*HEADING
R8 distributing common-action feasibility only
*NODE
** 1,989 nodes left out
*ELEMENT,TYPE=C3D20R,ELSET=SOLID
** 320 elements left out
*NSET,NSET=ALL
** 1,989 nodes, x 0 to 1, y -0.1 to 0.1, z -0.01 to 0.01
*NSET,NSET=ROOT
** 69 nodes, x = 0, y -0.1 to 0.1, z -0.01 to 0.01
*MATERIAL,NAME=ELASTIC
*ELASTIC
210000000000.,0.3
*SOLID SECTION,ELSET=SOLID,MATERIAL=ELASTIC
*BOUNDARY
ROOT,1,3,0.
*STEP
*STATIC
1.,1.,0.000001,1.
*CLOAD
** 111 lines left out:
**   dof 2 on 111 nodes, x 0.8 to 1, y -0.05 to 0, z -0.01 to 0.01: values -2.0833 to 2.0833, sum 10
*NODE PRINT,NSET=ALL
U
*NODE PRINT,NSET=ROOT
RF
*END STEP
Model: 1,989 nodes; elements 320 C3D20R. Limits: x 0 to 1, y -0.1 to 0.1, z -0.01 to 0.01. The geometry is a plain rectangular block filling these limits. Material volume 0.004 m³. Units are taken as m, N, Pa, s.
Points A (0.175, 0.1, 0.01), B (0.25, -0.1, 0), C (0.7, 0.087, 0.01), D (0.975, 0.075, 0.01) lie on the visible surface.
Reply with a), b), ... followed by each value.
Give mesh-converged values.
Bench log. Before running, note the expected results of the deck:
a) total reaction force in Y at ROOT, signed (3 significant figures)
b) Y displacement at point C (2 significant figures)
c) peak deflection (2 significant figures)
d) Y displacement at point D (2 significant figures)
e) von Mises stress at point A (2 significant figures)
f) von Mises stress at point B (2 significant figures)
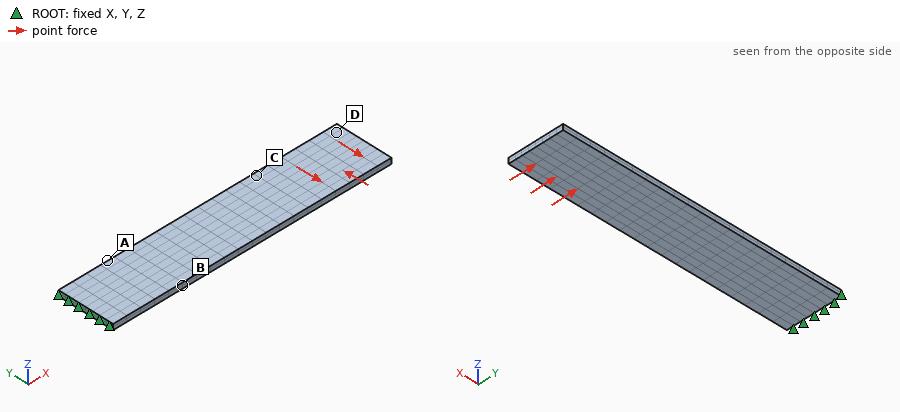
a) -10.0 N
b) 6.9e-07 m
c) 1.6e-06 m
d) 1.1e-06 m
e) 53000 Pa
f) 54000 Pa
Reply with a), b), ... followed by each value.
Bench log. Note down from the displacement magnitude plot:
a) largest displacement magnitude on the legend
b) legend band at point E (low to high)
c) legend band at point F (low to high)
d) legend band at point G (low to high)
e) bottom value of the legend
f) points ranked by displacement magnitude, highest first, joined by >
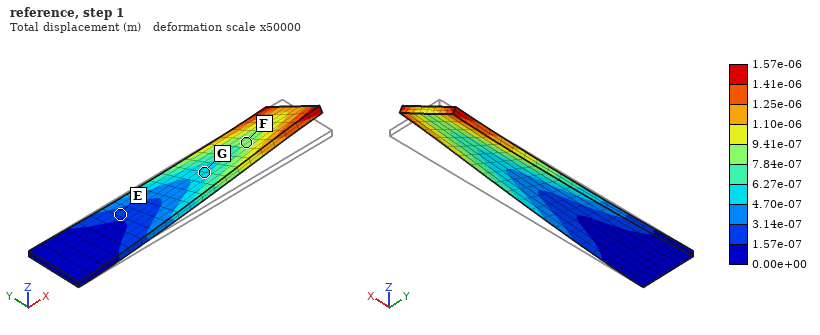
a) 1.57e-06 m
b) 1.57e-07 to 3.14e-07 m
c) 7.84e-07 to 9.41e-07 m
d) 4.70e-07 to 6.27e-07 m
e) 0.00e+00 m
f) F > G > E
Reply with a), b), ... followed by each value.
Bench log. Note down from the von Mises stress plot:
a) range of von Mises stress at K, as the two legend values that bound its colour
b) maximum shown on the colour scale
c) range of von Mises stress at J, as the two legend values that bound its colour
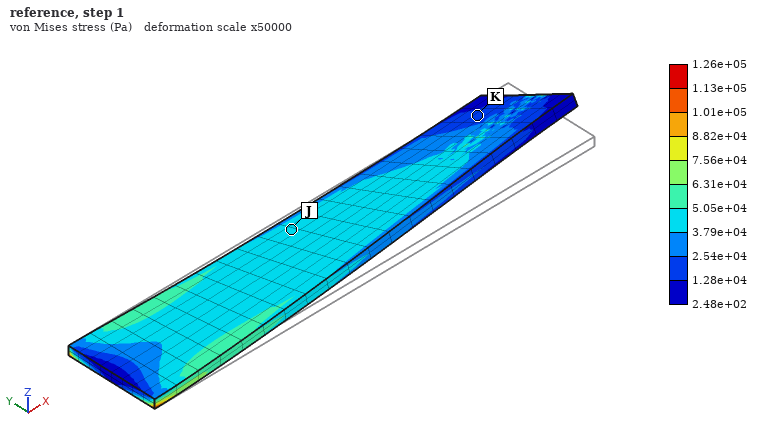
a) 1.28e+04 to 2.54e+04 Pa
b) 1.26e+05 Pa
c) 3.79e+04 to 5.05e+04 Pa
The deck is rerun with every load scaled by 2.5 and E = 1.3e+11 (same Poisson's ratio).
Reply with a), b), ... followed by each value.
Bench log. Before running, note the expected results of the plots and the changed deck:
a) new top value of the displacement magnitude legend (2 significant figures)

a) 6.3e-06 m
